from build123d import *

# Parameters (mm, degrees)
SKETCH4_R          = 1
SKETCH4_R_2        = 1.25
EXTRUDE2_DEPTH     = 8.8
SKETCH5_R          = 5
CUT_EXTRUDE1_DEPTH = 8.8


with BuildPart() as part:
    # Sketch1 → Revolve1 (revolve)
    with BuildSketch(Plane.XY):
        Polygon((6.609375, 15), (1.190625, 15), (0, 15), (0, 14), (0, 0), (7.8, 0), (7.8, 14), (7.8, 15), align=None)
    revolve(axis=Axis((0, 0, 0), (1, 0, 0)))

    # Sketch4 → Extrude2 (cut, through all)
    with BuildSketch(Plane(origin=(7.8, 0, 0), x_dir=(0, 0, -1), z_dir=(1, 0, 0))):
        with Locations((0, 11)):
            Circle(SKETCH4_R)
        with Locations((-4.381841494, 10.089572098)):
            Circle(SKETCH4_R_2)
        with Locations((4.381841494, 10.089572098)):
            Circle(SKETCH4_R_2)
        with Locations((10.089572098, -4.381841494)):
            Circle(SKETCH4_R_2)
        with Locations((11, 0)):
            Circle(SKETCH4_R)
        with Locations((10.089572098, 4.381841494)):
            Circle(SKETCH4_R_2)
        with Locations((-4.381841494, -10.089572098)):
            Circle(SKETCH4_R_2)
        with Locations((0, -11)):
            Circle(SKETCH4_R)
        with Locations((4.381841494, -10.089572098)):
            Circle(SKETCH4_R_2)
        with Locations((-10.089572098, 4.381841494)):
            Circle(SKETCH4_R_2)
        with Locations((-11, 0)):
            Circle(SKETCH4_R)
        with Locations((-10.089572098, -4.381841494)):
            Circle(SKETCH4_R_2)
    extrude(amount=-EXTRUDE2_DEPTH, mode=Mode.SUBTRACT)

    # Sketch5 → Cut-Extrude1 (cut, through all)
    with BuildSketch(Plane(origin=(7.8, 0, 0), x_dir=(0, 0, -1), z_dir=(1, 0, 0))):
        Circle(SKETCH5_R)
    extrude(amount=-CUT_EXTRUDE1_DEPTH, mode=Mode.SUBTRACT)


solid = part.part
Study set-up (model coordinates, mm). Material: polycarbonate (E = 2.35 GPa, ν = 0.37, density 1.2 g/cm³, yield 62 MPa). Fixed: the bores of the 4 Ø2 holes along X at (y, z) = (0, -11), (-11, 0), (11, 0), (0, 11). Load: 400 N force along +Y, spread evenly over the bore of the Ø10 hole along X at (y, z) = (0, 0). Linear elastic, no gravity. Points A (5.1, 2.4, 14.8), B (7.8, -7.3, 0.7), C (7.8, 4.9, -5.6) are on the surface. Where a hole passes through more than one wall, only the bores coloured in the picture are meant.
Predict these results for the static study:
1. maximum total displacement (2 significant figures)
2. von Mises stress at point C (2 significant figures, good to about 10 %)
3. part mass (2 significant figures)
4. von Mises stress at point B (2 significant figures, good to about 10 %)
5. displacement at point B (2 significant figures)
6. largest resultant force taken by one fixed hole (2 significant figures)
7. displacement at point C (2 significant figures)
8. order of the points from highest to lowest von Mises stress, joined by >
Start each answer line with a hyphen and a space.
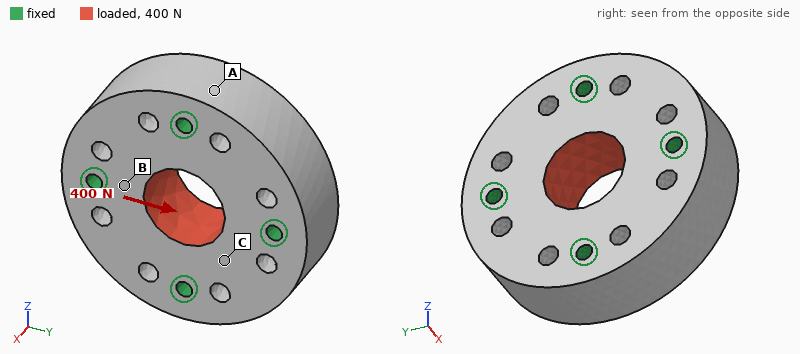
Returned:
- 9.2 µm
- 1.4 MPa
- 5.4 g
- 2.6 MPa
- 3.8 µm
- 120 N
- 6.8 µm
- B > C > A
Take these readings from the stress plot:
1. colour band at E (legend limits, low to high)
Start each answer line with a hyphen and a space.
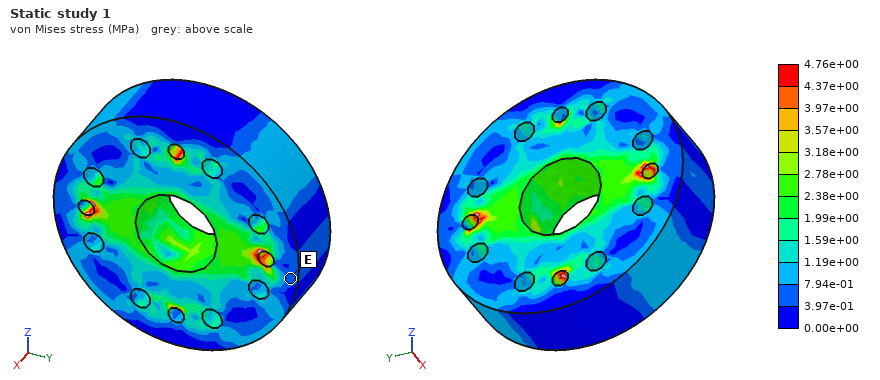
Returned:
- 3.97e-01 to 7.94e-01 MPa
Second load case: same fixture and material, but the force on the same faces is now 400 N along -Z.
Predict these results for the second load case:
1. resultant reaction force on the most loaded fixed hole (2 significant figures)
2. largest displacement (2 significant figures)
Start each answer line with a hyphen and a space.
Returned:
- 120 N
- 9.2 µm
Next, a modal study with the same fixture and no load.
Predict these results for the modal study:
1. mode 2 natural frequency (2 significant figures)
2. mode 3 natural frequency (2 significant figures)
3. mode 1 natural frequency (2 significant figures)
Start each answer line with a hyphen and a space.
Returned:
- 16 kHz
- 16 kHz
- 15 kHz
